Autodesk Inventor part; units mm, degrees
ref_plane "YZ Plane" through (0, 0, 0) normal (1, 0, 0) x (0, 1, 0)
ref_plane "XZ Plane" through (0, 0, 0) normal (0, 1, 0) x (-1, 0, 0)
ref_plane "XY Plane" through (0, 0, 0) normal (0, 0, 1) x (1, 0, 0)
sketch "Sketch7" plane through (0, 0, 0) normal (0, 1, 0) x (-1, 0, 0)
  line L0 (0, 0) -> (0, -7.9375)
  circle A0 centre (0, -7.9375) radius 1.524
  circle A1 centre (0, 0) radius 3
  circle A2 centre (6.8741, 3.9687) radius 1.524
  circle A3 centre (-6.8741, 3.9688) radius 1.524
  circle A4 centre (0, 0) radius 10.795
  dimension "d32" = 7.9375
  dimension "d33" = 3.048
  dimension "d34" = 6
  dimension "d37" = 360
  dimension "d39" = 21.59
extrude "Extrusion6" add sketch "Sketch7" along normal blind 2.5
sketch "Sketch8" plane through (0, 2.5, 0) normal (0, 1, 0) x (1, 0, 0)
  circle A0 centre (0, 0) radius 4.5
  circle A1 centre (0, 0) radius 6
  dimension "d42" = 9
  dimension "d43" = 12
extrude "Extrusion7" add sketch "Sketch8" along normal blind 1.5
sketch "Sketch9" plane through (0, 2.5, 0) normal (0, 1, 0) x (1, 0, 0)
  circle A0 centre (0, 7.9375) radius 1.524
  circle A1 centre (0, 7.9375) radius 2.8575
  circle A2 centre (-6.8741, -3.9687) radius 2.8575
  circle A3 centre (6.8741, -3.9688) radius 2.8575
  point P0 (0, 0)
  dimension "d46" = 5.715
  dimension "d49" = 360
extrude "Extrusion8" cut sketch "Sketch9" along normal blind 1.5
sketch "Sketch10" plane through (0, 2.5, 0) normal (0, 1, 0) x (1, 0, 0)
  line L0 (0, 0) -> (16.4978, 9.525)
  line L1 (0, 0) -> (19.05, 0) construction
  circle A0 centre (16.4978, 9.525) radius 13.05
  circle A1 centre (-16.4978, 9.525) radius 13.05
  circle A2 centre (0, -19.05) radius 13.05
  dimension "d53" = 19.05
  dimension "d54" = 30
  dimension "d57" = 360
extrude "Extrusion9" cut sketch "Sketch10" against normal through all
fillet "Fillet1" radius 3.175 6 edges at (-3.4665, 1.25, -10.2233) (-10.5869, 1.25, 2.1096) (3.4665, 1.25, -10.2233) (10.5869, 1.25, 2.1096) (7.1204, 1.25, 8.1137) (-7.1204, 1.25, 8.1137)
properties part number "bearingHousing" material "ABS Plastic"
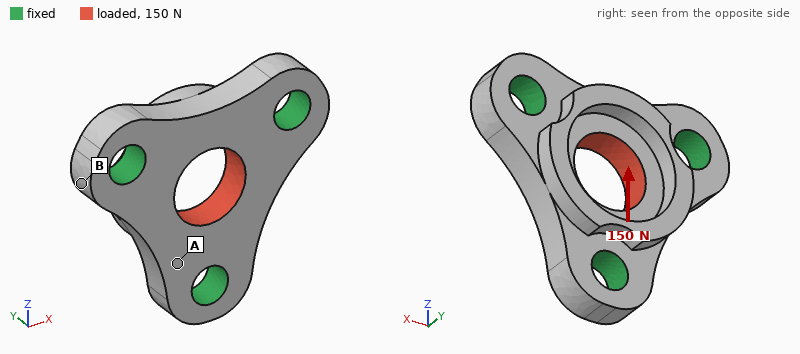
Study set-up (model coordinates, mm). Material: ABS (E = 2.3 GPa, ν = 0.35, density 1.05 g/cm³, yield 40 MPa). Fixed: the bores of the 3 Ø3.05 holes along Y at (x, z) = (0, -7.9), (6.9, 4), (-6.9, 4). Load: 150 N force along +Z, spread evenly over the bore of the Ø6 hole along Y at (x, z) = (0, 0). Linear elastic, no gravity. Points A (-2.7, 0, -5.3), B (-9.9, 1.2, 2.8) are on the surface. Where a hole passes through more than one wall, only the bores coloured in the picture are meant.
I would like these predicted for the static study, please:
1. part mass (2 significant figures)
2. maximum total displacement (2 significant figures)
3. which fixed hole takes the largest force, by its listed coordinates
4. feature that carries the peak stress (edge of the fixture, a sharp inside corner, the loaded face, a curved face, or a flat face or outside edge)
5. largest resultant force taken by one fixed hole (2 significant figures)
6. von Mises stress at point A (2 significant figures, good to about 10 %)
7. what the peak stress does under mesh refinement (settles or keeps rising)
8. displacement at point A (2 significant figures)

0.51 g
24 µm
(0, -7.9)
edge of the fixture
57 N
2.9 MPa
keeps rising
5.5 µm
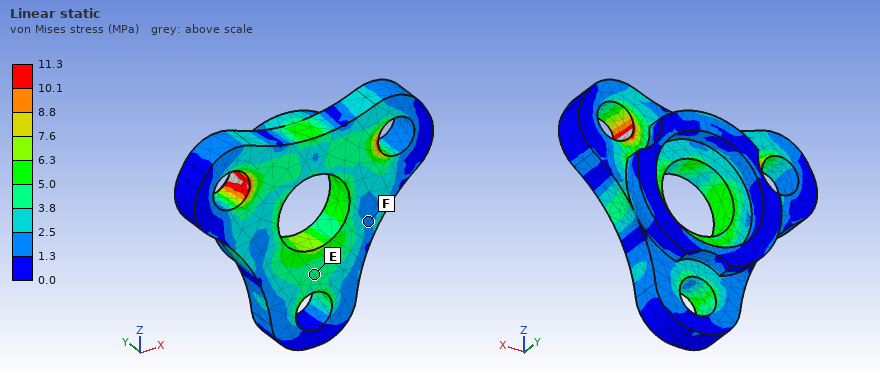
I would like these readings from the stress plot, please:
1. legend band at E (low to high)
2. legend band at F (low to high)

3.8 to 5.0 MPa
1.3 to 2.5 MPa
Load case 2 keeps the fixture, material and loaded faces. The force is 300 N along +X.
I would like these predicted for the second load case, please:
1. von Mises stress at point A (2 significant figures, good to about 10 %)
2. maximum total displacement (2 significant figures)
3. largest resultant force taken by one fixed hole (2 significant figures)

8.4 MPa
43 µm
110 N
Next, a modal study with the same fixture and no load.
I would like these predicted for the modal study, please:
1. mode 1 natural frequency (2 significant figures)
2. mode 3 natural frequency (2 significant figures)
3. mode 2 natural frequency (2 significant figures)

24 kHz
24 kHz
24 kHz
